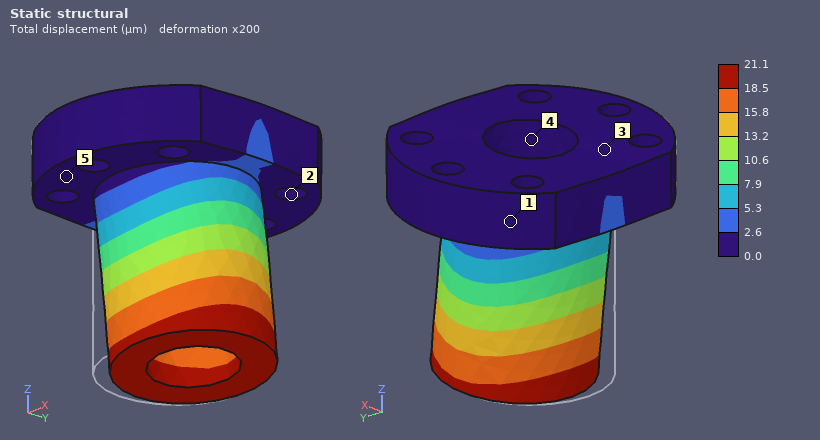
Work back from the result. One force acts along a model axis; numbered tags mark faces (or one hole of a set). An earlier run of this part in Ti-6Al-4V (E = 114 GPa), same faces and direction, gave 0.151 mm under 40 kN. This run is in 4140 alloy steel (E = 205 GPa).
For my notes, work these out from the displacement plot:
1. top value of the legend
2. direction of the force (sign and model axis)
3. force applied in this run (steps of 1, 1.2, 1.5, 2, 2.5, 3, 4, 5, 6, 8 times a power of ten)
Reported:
21.1 µm
+X
10 kN
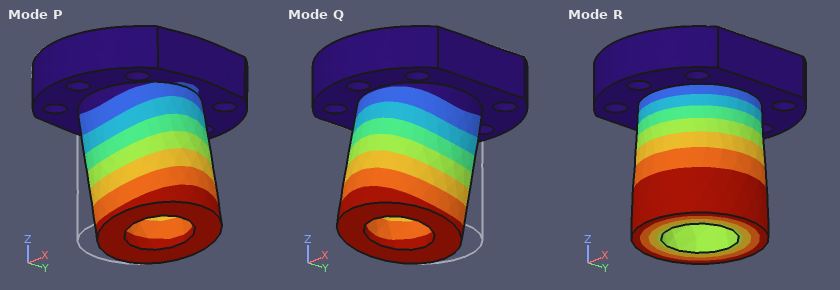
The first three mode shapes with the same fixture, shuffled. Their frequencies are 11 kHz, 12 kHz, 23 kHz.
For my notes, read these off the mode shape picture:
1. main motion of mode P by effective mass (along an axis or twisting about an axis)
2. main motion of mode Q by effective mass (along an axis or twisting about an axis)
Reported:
along X
along Y
